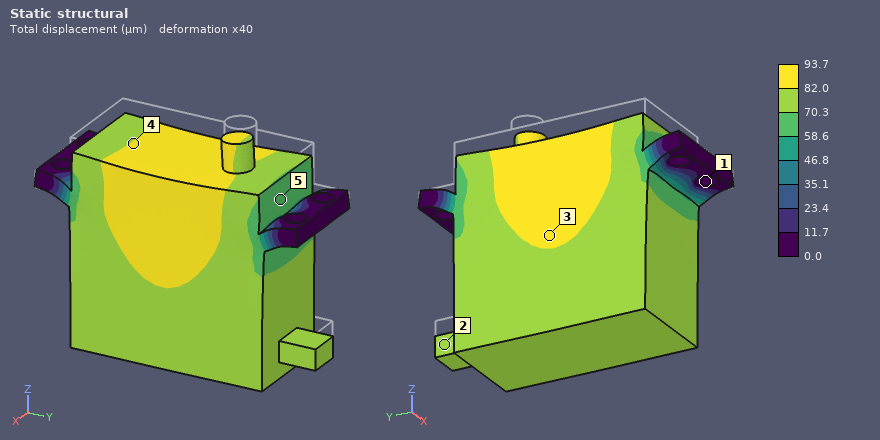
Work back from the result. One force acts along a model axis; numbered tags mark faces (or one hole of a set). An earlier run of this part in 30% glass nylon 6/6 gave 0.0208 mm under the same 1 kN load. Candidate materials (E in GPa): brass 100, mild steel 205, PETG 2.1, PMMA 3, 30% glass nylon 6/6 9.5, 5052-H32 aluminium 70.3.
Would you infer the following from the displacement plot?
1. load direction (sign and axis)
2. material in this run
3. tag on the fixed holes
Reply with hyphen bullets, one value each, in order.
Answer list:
- -Z
- PETG
- 1
